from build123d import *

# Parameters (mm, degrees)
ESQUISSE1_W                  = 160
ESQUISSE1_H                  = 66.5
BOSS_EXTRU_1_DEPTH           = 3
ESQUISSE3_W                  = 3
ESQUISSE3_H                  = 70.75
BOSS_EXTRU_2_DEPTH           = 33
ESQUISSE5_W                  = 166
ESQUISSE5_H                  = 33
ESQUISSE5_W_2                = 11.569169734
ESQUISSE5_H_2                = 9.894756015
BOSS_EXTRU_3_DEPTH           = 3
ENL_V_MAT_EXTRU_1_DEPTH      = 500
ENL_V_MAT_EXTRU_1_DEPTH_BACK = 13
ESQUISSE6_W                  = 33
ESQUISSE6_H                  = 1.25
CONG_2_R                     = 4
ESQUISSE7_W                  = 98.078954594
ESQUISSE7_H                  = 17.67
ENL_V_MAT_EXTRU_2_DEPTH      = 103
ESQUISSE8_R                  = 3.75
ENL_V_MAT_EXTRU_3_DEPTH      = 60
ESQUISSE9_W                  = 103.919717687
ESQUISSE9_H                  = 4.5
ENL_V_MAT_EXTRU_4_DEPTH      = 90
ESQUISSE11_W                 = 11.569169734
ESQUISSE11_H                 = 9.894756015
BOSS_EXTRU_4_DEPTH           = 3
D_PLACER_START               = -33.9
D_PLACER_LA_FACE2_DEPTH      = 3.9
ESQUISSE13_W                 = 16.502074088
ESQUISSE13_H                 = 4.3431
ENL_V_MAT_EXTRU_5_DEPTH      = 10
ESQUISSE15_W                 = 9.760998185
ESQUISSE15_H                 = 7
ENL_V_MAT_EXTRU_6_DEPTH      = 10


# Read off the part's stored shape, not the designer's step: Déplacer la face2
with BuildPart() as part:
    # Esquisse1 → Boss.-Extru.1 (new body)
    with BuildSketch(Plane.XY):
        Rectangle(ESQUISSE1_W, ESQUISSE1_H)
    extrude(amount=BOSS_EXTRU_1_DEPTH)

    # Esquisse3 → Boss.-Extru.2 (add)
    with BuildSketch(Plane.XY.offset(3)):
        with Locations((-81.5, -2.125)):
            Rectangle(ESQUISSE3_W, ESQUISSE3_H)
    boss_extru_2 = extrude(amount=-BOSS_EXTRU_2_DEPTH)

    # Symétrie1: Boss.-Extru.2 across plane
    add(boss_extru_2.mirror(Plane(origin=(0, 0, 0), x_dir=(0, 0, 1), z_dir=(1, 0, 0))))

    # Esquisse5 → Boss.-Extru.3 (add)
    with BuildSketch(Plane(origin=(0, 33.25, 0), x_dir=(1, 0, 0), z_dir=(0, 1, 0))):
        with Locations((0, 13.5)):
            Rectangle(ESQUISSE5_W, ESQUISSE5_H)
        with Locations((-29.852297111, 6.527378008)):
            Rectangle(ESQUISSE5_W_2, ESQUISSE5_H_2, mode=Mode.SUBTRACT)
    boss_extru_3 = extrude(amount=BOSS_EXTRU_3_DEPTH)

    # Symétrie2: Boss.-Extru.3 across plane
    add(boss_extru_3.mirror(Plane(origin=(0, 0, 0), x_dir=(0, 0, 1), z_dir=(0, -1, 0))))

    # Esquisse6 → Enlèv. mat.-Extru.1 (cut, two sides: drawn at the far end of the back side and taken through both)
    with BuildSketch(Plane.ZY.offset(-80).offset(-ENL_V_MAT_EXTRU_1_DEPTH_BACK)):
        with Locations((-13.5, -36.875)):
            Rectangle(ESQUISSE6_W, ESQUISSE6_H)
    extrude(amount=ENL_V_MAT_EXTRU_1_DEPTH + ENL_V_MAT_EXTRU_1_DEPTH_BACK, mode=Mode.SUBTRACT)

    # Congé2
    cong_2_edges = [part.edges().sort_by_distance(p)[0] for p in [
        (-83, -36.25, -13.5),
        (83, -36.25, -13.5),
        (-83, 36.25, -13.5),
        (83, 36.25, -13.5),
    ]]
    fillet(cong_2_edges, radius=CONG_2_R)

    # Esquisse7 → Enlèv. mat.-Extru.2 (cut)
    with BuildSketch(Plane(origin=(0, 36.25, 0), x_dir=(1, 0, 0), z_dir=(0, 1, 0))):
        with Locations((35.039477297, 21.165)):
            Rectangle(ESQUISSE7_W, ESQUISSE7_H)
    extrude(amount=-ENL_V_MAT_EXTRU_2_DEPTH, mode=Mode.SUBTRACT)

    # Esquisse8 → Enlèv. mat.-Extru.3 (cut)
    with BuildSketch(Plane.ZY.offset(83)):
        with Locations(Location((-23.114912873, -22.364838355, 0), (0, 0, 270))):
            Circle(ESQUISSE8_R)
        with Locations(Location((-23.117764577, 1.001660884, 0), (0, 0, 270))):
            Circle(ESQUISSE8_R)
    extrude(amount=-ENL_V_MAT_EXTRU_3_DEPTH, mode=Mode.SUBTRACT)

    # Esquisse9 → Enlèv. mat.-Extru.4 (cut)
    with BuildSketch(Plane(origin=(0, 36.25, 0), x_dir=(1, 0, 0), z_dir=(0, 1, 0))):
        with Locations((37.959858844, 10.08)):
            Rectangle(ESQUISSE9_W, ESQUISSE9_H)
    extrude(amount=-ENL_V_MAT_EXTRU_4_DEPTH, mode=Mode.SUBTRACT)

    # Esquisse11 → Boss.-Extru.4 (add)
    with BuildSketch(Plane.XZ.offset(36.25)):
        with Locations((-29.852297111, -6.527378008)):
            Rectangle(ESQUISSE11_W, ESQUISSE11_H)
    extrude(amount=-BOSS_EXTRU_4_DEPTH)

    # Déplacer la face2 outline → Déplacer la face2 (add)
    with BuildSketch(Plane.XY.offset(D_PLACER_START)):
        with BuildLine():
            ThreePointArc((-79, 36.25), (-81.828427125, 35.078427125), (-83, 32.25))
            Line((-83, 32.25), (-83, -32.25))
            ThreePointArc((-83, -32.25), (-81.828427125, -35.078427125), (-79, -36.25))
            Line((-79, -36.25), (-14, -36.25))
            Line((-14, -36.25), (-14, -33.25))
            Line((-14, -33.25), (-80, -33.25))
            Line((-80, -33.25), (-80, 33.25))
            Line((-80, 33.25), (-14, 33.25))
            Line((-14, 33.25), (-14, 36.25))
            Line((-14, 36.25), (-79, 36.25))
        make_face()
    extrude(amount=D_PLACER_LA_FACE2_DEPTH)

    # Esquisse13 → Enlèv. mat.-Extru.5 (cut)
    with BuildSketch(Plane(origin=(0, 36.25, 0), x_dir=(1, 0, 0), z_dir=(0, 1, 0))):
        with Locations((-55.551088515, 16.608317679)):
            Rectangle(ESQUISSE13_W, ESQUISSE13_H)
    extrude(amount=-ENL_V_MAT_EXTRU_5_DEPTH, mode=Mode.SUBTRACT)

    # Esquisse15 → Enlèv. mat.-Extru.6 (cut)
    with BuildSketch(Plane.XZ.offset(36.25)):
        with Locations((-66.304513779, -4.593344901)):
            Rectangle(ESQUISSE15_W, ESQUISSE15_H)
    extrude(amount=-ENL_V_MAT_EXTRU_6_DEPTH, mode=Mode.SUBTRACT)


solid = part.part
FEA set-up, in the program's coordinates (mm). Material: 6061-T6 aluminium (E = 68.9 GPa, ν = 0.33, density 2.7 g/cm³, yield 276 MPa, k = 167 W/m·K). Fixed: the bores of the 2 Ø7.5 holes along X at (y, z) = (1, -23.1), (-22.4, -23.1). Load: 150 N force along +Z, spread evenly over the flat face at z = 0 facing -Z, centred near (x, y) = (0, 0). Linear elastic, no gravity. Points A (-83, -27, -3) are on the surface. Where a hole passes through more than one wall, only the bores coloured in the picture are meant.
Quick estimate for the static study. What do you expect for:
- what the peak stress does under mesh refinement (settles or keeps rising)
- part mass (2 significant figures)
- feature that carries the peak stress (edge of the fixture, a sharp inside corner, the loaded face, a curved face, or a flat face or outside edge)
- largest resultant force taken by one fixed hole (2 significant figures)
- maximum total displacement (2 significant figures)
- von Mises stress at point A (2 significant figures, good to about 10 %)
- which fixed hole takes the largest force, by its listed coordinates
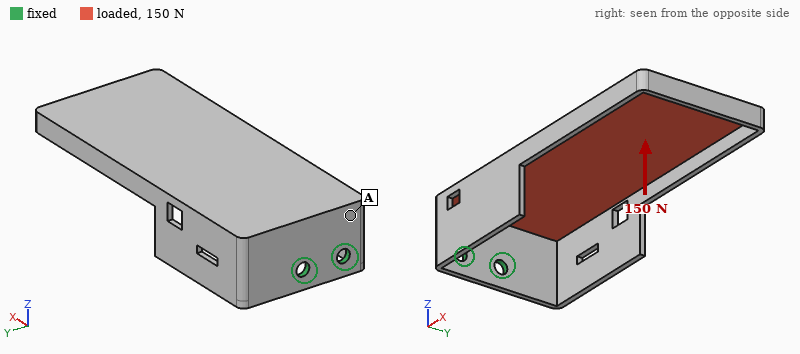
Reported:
keeps rising
170 g
edge of the fixture
140 N
1.7 mm
17 MPa
(1, -23.1)
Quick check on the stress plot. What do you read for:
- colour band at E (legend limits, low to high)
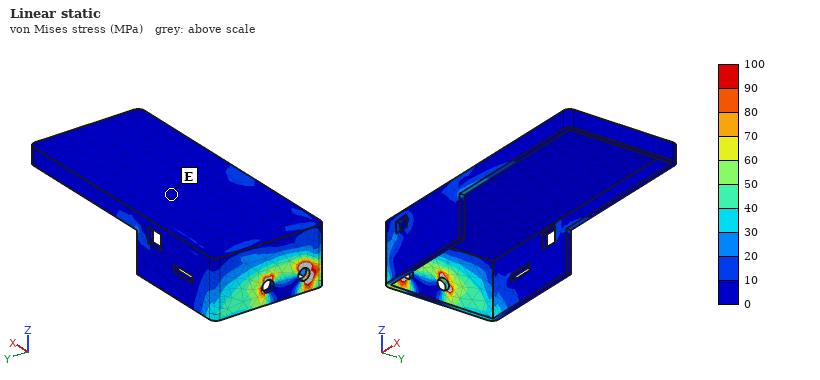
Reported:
0 to 10 MPa
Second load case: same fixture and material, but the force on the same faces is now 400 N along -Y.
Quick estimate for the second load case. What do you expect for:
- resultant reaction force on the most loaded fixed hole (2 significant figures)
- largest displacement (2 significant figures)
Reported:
890 N
2.1 mm
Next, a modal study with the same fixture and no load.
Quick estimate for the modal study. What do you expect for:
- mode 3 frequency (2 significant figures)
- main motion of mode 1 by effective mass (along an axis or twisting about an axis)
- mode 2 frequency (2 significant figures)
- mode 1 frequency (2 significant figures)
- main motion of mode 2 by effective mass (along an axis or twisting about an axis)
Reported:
590 Hz
along Z
230 Hz
160 Hz
along Y
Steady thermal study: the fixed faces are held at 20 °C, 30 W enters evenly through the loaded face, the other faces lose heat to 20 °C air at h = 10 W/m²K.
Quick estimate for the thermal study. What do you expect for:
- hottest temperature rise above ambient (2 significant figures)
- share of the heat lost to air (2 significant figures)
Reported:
44 K
28 %
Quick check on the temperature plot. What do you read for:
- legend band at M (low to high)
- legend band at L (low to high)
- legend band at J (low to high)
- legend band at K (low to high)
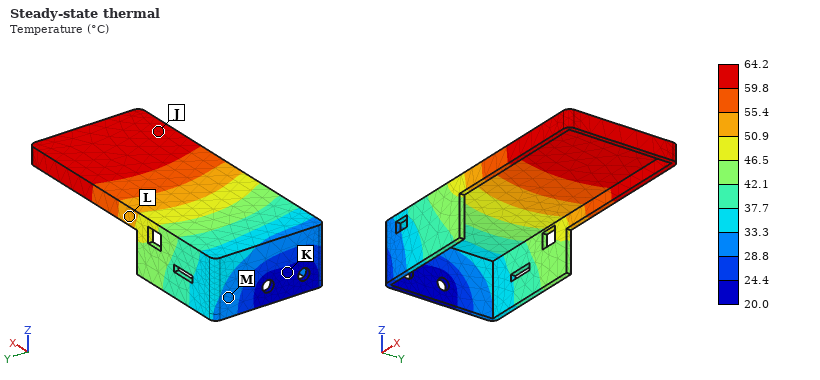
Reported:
28.8 to 33.3 °C
50.9 to 55.4 °C
59.8 to 64.2 °C
20.0 to 24.4 °C
